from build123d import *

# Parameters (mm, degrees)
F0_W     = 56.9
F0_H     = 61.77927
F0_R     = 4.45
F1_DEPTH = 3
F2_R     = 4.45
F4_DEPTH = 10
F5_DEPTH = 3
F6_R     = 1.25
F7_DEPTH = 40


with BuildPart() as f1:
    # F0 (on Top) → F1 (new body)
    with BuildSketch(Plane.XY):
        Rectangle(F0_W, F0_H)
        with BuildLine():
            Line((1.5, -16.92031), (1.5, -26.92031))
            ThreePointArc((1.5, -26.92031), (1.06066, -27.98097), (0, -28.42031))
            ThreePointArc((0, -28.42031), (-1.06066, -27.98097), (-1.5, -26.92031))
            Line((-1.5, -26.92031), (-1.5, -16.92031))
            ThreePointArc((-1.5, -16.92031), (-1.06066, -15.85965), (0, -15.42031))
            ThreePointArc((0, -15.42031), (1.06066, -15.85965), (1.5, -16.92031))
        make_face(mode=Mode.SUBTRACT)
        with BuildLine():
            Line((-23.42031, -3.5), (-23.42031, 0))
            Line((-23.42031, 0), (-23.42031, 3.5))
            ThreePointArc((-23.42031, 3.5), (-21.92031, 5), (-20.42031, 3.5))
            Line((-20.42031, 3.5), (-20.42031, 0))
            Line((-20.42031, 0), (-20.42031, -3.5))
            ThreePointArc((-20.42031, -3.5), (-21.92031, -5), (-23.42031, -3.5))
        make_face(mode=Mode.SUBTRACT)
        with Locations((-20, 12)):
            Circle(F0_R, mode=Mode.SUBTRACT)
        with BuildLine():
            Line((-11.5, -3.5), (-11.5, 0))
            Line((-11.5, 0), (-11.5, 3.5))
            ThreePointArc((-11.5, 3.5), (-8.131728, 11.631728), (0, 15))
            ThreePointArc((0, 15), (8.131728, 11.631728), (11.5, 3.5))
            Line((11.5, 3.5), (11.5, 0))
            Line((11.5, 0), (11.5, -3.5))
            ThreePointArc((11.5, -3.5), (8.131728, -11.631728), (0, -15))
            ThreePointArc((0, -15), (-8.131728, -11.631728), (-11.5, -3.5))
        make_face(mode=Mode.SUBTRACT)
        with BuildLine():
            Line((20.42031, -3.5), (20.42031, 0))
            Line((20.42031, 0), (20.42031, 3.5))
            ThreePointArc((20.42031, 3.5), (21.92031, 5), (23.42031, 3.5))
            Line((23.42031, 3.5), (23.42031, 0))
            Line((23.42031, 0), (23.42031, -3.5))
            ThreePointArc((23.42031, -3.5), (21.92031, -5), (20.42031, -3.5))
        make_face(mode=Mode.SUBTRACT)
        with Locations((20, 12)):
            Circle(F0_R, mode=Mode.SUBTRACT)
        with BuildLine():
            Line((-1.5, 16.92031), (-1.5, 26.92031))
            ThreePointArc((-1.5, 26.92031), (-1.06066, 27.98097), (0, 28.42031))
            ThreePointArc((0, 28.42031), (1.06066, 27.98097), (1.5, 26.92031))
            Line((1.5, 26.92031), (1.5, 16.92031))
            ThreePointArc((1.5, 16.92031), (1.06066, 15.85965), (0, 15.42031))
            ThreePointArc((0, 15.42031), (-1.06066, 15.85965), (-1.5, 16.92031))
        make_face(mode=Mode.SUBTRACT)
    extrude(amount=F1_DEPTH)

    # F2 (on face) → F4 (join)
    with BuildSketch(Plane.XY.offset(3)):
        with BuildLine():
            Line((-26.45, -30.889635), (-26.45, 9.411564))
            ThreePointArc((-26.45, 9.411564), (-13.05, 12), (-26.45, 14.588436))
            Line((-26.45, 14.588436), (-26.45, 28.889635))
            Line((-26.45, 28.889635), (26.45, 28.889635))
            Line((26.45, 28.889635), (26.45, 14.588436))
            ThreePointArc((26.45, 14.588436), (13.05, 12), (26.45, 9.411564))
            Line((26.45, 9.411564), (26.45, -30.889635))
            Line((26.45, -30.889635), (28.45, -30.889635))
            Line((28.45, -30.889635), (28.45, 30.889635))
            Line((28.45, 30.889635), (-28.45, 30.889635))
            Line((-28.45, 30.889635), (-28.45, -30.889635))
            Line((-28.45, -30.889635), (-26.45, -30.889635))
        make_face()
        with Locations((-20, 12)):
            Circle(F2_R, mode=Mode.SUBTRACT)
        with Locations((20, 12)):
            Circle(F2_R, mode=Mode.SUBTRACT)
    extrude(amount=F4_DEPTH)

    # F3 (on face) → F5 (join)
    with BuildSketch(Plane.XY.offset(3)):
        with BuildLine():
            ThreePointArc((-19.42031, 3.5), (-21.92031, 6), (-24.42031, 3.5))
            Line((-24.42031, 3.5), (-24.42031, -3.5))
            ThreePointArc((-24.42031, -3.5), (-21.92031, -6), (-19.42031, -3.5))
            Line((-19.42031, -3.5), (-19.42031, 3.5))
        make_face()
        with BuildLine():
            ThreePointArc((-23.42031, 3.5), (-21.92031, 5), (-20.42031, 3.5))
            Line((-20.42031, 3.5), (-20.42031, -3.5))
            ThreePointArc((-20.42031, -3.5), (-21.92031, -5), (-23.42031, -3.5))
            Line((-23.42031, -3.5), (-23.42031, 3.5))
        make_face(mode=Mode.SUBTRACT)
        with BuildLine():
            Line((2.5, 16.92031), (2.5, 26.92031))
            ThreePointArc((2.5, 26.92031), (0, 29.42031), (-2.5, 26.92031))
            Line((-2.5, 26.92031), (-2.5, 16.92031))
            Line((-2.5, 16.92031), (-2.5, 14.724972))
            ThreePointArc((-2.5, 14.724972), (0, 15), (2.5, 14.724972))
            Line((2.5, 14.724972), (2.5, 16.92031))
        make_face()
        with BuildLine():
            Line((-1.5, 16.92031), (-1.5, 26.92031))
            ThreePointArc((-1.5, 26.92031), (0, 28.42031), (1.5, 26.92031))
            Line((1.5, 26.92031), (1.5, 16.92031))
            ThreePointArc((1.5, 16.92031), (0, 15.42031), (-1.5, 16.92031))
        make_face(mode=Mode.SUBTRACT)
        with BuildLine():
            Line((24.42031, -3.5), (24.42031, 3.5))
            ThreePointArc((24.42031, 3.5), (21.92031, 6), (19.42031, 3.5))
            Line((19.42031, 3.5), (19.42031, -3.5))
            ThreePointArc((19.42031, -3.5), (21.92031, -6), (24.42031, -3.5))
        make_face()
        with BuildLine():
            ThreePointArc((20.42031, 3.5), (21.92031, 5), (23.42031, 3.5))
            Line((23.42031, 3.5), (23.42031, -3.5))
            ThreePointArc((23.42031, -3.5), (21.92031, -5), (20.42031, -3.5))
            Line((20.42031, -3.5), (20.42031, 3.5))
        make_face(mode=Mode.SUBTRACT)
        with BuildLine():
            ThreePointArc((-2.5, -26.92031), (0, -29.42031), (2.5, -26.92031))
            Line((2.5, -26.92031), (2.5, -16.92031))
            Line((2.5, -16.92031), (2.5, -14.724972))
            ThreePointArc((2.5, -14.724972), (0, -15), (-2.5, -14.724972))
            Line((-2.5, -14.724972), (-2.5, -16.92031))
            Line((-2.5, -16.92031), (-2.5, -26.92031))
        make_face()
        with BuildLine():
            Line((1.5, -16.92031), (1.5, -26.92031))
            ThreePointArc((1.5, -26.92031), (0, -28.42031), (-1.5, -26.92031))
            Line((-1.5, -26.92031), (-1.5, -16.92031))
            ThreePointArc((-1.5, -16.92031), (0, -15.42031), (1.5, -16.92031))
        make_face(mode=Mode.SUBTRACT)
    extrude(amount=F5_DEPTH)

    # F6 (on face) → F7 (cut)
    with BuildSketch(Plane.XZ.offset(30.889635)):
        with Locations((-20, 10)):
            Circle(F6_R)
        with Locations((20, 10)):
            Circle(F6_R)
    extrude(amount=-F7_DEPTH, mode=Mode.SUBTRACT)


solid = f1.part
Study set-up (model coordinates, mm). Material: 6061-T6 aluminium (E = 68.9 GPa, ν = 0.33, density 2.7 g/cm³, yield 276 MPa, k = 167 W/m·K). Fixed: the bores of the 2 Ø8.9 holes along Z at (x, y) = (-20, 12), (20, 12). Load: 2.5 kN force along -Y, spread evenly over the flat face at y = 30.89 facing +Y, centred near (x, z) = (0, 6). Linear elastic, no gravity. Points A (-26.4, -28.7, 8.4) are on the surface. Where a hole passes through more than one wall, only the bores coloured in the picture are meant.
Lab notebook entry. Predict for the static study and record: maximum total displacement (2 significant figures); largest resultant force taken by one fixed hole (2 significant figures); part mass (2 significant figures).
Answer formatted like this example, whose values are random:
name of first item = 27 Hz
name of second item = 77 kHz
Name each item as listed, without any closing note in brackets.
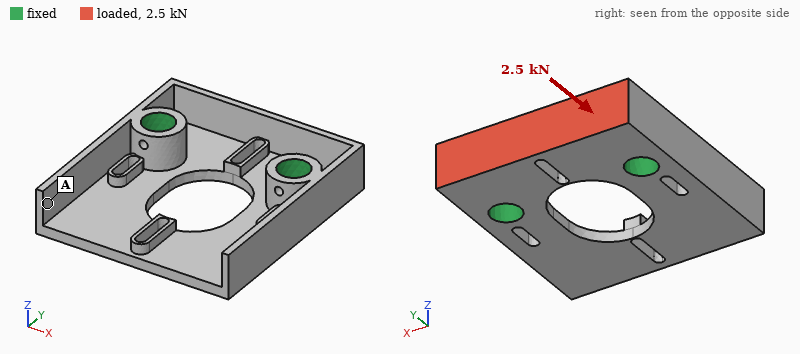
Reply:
maximum total displacement = 0.18 mm
largest resultant force taken by one fixed hole = 1.3 kN
part mass = 37 g
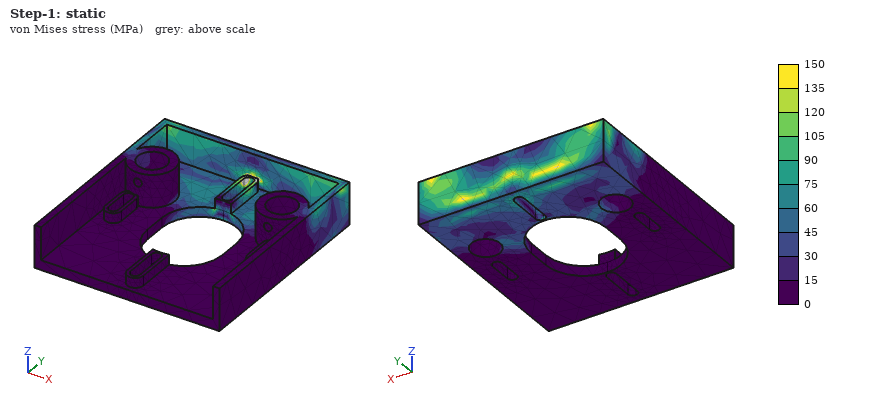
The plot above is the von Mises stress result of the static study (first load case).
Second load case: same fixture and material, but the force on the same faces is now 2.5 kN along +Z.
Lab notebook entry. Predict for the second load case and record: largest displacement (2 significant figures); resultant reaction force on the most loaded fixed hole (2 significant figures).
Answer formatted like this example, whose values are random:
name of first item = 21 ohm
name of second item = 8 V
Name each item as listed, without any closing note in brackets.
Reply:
largest displacement = 0.24 mm
resultant reaction force on the most loaded fixed hole = 1.3 kN
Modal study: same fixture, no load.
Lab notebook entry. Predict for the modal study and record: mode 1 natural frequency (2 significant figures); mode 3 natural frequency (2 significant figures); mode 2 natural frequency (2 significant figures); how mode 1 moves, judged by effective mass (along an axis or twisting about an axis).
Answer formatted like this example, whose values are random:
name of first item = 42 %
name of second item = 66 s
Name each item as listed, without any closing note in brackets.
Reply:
mode 1 natural frequency = 2800 Hz
mode 3 natural frequency = 6400 Hz
mode 2 natural frequency = 4900 Hz
how mode 1 moves, judged by effective mass = along Z
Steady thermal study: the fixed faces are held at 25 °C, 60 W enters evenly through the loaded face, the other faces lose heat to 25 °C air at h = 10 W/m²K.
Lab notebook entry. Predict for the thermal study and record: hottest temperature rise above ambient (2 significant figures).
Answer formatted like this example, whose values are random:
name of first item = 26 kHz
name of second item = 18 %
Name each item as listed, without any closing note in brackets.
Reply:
hottest temperature rise above ambient = 46 K
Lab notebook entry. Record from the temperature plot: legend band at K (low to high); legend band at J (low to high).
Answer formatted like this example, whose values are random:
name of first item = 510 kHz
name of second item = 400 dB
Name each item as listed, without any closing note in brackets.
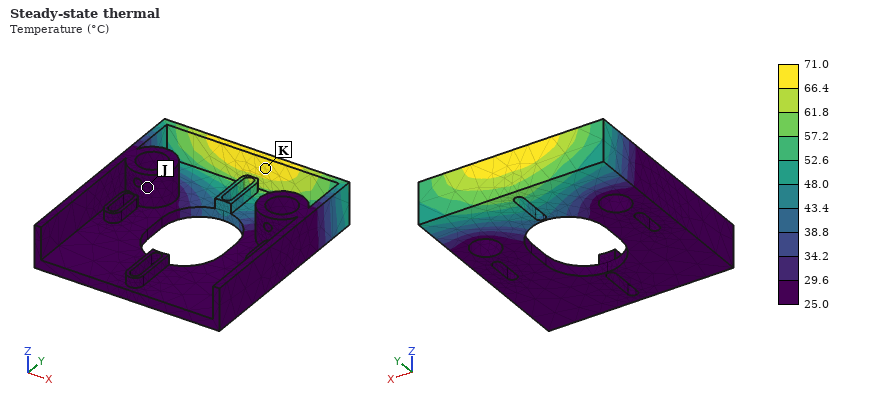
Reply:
legend band at K = 66.4 to 71.0 °C
legend band at J = 25.0 to 29.6 °C
